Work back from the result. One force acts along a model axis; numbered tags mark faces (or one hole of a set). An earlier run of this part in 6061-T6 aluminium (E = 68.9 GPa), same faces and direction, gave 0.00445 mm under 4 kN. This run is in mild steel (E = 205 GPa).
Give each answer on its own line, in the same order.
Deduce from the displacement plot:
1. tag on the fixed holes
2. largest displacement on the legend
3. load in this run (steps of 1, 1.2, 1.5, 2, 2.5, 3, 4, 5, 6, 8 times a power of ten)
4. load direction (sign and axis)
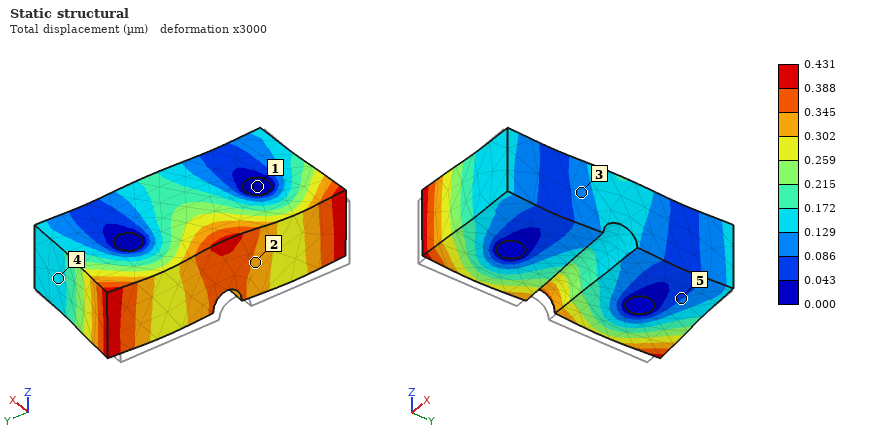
1
0.431 µm
1.2 kN
+X
